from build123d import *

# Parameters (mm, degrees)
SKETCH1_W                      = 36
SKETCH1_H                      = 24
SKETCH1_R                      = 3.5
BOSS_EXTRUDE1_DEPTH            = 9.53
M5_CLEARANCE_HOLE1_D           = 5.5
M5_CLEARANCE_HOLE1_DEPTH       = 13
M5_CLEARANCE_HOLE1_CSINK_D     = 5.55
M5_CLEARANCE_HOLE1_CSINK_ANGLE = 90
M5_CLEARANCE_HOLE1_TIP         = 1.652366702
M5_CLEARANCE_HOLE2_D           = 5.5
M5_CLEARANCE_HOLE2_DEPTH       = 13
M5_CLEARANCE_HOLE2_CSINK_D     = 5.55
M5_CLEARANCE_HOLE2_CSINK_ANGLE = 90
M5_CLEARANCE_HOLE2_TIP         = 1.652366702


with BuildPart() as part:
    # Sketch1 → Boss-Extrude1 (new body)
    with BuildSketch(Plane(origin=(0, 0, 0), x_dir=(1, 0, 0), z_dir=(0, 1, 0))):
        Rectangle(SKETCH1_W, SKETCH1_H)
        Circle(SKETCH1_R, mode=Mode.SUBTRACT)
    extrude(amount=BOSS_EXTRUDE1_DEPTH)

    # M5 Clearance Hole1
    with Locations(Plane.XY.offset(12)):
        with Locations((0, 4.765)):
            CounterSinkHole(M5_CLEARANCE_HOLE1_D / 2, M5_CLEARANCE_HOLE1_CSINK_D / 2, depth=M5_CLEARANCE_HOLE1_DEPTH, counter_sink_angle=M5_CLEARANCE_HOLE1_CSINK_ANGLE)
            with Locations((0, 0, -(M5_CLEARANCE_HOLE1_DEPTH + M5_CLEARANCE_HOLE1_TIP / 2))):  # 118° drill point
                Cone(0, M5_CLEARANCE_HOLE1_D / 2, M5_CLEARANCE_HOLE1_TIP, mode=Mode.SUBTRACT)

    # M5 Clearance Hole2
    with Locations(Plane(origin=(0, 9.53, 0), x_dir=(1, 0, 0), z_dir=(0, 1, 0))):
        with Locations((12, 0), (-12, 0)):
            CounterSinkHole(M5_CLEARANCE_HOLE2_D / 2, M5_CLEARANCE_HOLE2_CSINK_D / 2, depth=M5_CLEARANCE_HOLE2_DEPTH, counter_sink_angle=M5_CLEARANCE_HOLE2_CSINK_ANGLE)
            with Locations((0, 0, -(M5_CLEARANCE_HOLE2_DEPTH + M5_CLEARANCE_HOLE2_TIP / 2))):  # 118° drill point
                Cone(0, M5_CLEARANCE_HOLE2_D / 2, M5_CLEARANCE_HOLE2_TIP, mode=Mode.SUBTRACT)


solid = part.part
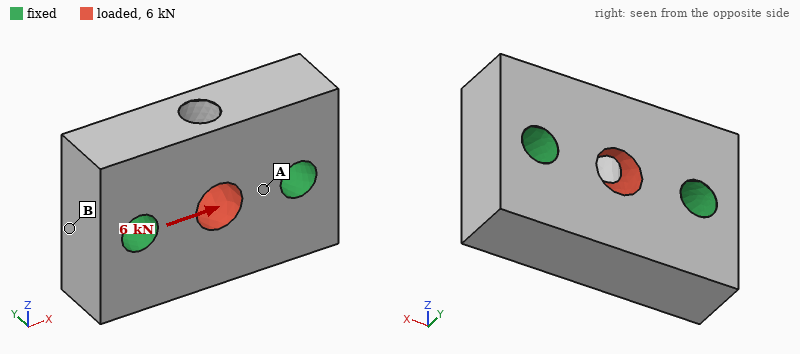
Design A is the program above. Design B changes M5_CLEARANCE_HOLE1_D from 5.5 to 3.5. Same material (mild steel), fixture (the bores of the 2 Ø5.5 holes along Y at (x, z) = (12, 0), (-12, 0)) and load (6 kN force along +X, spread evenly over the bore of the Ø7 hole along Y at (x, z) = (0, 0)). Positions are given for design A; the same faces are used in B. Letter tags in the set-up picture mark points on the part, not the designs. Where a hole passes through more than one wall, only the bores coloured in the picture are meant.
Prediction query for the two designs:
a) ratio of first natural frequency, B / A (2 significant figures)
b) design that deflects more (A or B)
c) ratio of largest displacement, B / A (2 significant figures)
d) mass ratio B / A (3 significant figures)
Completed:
0.99
A
0.91
1.02
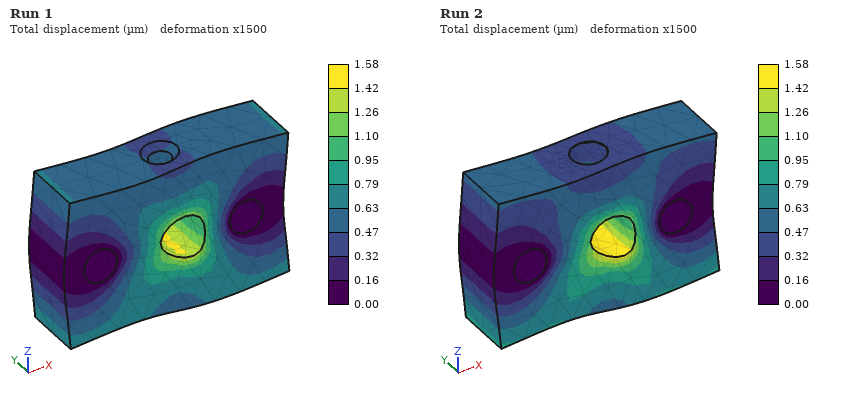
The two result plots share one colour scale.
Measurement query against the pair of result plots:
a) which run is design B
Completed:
Run 1
